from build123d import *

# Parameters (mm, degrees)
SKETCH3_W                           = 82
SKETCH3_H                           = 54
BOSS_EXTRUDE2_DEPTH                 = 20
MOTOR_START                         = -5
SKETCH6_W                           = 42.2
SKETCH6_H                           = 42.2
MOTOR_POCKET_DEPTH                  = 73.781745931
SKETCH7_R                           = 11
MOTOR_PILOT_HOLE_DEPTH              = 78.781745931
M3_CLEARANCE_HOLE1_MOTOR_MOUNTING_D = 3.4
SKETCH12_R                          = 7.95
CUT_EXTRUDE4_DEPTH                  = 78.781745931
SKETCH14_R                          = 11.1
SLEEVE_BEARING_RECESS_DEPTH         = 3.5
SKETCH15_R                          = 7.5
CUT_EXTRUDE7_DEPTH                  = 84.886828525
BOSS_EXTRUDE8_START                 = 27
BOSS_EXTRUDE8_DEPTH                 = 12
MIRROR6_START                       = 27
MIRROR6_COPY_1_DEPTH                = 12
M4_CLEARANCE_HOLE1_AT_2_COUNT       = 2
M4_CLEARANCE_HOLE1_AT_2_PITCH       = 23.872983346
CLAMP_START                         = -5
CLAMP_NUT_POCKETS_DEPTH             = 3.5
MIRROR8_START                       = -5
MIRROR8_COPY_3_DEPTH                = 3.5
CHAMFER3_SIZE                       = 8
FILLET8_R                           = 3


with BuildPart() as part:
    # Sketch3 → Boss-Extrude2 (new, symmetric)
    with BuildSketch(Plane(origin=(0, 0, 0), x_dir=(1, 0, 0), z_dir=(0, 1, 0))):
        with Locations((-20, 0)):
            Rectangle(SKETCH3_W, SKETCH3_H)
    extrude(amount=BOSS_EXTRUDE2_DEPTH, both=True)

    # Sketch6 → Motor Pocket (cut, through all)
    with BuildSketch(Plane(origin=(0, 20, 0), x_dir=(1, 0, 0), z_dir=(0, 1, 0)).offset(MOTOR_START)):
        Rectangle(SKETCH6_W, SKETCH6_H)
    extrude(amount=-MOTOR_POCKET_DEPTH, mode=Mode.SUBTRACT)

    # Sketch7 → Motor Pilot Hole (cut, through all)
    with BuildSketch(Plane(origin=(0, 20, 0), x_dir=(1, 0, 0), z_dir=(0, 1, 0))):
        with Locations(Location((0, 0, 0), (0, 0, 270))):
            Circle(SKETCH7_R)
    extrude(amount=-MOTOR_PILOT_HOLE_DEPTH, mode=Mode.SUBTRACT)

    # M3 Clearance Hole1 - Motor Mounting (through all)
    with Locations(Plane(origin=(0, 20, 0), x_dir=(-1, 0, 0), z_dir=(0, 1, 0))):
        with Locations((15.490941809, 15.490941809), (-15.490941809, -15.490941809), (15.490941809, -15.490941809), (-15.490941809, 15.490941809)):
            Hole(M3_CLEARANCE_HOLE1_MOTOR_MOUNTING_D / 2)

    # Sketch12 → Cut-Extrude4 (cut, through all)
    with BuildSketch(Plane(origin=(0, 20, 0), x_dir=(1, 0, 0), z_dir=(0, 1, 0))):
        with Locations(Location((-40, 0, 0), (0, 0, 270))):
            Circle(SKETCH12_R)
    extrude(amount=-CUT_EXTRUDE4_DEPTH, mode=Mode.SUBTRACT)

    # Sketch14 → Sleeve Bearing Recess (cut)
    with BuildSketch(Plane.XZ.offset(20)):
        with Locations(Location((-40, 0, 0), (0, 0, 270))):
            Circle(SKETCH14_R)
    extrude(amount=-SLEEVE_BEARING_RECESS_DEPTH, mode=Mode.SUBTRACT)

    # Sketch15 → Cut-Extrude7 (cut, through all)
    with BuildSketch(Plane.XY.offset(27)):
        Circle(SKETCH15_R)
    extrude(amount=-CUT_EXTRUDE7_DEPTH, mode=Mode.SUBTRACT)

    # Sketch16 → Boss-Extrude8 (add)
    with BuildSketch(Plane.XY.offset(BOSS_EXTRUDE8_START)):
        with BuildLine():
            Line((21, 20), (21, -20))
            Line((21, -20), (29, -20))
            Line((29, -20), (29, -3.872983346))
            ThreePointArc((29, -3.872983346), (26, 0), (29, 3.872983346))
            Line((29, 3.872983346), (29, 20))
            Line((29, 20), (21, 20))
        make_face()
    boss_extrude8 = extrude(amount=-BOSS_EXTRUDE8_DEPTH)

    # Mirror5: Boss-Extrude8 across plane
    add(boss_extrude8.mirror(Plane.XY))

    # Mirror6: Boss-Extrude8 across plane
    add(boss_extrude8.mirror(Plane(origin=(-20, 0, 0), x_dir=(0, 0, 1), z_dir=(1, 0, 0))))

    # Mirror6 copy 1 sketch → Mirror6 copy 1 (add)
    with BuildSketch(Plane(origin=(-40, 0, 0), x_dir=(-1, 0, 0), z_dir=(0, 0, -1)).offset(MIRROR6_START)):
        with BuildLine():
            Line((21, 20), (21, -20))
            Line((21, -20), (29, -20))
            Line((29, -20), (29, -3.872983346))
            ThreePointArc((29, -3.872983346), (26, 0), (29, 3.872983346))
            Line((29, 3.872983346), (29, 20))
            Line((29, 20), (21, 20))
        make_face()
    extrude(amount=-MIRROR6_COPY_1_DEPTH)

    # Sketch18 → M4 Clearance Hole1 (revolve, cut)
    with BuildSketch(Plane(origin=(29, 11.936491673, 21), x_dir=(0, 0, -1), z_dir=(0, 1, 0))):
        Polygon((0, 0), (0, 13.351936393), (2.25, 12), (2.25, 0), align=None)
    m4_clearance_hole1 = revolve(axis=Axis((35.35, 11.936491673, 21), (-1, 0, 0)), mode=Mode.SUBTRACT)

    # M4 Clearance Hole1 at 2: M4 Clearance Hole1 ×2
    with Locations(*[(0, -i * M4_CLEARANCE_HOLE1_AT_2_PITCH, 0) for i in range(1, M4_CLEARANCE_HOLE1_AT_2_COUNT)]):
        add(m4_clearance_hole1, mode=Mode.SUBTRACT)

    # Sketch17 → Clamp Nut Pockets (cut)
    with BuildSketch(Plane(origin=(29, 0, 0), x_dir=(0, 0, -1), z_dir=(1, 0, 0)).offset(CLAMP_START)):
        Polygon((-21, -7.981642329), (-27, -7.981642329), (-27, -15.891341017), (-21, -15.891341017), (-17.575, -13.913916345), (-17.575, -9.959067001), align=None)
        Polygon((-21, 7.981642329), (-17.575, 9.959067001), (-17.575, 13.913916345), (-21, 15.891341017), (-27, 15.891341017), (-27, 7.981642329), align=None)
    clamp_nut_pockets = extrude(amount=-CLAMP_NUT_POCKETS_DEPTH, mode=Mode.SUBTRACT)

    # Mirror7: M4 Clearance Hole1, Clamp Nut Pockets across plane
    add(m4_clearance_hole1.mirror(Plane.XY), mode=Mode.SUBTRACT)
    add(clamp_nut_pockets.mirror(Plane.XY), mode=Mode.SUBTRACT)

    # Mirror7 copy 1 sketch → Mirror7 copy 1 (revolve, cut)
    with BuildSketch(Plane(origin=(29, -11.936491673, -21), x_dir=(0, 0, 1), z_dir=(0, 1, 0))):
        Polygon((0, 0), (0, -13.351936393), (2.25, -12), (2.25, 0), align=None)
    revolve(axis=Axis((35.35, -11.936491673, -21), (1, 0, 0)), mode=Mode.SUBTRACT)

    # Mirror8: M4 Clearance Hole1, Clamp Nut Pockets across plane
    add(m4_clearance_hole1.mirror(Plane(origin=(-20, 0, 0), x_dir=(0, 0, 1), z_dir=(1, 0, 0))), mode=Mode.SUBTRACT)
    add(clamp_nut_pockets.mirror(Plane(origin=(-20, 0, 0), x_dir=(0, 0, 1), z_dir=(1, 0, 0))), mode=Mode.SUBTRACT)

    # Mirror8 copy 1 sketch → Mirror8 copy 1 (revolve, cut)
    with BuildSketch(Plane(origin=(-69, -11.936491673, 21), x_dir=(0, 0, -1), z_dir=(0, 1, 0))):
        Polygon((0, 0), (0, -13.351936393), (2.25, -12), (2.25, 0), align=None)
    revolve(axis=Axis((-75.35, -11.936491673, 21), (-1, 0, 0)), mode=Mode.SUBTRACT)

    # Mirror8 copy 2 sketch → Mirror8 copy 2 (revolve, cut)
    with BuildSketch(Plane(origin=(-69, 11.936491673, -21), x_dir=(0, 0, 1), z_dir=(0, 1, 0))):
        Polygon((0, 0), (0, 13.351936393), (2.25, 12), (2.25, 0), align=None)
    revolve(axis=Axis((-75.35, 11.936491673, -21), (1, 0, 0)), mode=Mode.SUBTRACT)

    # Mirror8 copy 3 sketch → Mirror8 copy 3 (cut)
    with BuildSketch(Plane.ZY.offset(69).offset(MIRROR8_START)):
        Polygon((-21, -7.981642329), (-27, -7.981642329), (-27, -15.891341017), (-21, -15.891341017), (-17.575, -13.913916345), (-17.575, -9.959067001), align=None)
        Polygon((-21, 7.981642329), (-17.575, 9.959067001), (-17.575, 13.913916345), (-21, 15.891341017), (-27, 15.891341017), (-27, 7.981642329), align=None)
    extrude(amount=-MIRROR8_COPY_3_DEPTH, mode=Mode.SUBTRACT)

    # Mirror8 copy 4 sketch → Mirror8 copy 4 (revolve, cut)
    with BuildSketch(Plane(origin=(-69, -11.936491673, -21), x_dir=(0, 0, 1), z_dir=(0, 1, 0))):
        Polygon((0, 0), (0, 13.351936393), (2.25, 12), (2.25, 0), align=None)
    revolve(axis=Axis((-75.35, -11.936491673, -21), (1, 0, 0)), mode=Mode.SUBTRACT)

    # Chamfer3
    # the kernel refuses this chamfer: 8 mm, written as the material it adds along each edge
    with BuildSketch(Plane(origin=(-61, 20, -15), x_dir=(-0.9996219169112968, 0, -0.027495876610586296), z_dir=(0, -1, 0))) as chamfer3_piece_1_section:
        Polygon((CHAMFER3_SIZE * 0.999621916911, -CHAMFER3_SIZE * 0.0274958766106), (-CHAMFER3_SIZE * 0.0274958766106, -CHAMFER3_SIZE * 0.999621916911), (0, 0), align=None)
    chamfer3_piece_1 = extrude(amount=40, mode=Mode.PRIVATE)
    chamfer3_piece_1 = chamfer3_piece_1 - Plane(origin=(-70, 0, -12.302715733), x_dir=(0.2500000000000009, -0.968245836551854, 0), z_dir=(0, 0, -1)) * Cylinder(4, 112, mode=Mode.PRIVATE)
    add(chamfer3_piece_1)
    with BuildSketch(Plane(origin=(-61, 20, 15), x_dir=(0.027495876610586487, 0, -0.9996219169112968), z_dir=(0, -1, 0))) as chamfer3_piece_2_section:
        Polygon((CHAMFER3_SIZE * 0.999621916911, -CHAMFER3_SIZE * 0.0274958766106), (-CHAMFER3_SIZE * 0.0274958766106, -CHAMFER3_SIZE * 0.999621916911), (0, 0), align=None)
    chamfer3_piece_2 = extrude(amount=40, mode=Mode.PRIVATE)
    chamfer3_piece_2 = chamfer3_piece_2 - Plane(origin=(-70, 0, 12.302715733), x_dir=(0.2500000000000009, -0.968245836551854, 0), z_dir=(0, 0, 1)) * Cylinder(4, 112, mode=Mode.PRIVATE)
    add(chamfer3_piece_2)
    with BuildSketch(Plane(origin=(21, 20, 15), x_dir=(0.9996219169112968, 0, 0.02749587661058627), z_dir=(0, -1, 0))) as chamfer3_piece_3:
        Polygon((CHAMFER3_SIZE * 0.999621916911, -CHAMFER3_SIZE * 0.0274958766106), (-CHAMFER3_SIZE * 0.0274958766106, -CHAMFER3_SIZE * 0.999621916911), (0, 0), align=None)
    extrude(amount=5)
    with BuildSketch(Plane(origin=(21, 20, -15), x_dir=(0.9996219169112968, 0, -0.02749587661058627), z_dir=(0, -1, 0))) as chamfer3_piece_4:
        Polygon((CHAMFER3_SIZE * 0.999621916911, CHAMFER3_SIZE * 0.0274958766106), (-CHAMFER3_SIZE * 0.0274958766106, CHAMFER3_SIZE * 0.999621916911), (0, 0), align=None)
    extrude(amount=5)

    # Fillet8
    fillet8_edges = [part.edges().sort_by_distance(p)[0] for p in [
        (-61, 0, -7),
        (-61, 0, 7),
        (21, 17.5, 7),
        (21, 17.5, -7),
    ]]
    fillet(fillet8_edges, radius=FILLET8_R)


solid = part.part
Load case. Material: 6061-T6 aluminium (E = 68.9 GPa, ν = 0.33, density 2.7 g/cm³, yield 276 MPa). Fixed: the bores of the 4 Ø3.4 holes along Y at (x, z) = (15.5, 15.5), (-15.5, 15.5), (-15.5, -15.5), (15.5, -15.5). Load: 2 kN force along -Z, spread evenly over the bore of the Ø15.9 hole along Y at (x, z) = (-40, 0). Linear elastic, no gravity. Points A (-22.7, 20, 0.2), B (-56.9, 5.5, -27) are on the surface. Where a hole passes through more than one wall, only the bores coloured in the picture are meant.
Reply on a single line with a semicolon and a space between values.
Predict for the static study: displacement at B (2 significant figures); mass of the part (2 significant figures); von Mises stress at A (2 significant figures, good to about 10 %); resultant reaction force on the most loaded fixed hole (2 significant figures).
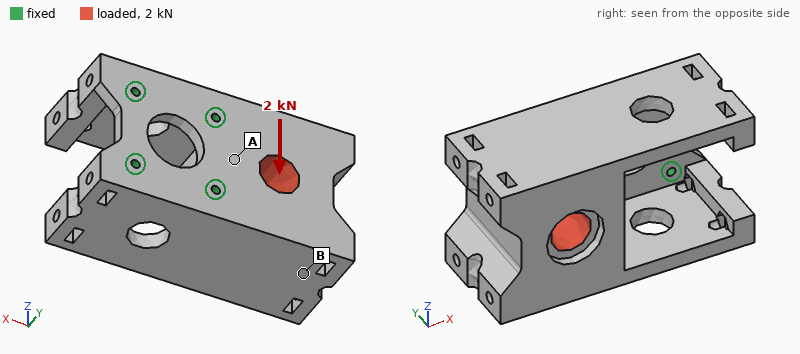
15 µm; 320 g; 8.3 MPa; 1.6 kN
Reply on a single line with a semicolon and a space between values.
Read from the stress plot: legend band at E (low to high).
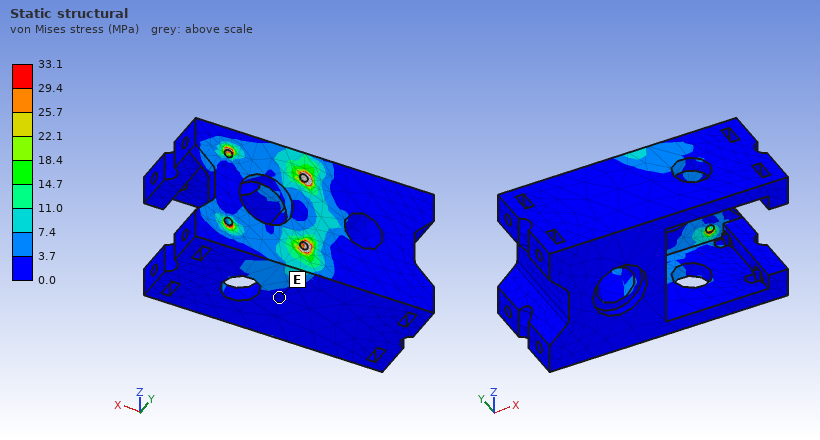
0.0 to 3.7 MPa
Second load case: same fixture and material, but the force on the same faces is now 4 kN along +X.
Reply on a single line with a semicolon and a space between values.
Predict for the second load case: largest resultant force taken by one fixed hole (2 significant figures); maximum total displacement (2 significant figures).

1.6 kN; 63 µm
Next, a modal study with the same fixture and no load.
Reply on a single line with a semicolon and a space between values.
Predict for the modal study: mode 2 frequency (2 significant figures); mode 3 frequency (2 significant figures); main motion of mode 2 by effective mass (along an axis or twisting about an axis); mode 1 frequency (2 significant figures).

3000 Hz; 4000 Hz; along Z; 2000 Hz
